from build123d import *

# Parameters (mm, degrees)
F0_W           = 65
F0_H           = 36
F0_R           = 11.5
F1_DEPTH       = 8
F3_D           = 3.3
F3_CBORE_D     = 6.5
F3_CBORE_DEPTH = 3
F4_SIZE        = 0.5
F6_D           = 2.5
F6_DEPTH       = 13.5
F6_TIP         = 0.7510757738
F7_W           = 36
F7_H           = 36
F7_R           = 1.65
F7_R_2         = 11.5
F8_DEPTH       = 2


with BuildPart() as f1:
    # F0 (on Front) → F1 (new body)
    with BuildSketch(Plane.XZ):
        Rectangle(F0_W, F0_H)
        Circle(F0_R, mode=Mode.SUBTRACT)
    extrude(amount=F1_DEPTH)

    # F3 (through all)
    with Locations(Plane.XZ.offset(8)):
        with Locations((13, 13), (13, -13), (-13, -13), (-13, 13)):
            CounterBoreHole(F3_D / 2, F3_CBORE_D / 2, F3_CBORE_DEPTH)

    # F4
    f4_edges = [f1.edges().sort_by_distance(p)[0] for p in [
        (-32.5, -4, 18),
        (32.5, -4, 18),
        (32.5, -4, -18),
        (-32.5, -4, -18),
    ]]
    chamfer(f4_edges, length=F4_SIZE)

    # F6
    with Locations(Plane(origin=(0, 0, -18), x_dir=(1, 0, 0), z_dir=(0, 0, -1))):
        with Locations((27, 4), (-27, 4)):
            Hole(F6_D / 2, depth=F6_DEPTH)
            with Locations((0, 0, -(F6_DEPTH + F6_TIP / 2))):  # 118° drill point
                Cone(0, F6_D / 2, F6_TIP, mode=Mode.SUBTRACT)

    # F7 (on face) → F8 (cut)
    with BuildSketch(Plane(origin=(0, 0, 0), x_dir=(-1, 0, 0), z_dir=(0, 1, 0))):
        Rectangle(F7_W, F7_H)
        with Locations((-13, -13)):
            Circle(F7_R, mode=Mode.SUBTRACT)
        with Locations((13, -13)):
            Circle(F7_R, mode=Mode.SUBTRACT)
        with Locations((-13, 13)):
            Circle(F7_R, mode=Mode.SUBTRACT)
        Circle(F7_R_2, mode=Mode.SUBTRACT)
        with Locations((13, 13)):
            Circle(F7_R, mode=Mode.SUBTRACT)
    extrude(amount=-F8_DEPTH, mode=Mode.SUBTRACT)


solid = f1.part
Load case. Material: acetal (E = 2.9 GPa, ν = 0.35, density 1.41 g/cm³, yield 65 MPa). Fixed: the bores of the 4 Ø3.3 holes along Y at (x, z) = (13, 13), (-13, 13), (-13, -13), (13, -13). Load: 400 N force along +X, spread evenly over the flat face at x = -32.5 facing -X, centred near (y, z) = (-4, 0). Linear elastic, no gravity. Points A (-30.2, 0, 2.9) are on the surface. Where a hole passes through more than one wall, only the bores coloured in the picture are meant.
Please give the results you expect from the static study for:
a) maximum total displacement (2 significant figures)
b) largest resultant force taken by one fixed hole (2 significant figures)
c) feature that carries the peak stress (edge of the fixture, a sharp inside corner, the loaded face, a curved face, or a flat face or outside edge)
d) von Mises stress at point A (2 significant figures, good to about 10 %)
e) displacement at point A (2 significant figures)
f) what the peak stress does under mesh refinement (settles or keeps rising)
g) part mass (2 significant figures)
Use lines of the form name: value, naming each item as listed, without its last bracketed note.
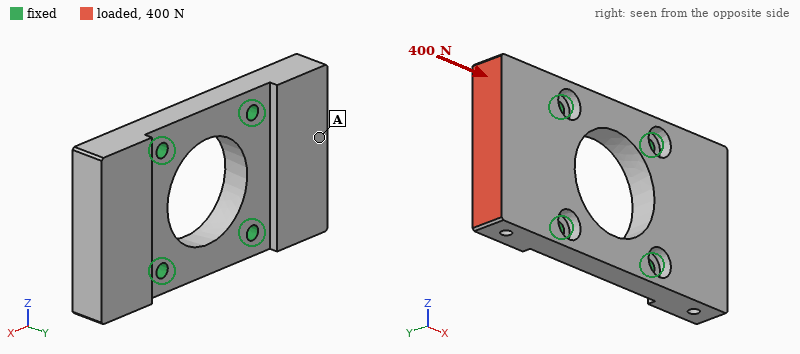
maximum total displacement: 22 µm
largest resultant force taken by one fixed hole: 190 N
feature that carries the peak stress: edge of the fixture
von Mises stress at point A: 1.2 MPa
displacement at point A: 20 µm
what the peak stress does under mesh refinement: keeps rising
part mass: 18 g
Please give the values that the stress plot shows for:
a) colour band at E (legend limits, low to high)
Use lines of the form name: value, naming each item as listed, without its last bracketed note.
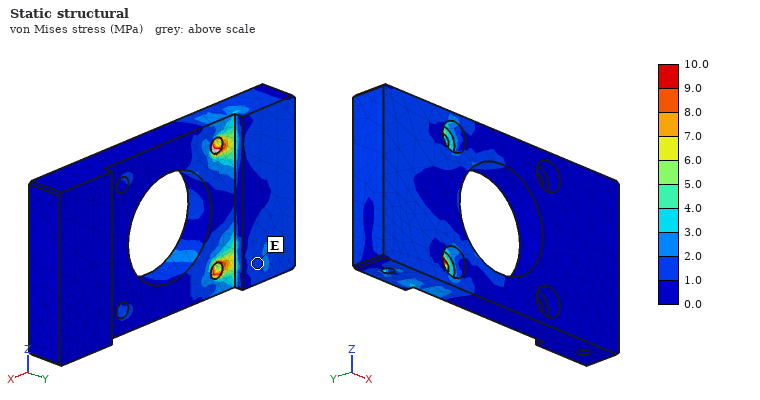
colour band at E: 1.0 to 2.0 MPa
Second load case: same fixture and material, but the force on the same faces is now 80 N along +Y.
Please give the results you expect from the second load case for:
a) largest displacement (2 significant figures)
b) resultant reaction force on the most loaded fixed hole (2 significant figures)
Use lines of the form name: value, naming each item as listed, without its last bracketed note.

largest displacement: 0.25 mm
resultant reaction force on the most loaded fixed hole: 62 N
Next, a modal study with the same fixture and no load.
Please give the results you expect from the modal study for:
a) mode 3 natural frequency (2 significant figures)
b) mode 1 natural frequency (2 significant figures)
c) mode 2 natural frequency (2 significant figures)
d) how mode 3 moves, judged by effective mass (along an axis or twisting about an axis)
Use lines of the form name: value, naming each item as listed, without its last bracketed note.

mode 3 natural frequency: 4500 Hz
mode 1 natural frequency: 1800 Hz
mode 2 natural frequency: 1900 Hz
how mode 3 moves, judged by effective mass: twisting about X
